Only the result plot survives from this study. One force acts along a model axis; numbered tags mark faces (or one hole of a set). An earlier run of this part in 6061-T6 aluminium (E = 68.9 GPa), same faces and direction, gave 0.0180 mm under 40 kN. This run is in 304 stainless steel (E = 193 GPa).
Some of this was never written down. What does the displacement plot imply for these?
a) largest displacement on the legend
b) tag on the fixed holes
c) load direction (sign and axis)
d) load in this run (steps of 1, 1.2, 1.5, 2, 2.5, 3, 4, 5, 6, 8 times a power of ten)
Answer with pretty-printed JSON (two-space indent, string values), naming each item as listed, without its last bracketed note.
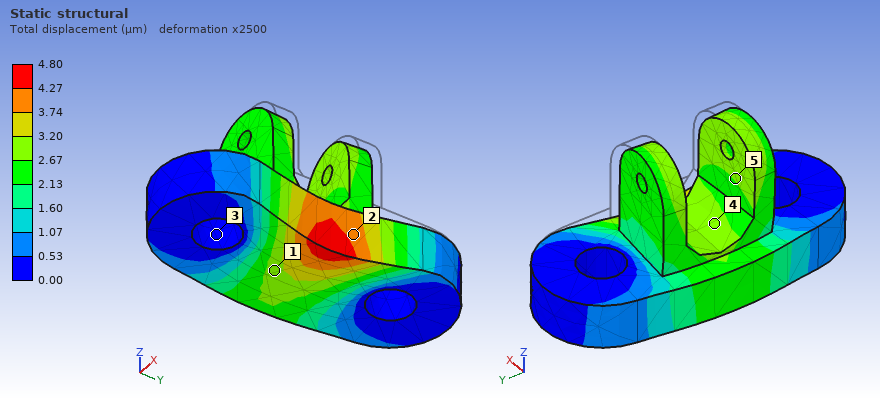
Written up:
{
  "largest displacement on the legend": "4.80 µm",
  "tag on the fixed holes": "3",
  "load direction": "-X",
  "load in this run": "30 kN"
}
